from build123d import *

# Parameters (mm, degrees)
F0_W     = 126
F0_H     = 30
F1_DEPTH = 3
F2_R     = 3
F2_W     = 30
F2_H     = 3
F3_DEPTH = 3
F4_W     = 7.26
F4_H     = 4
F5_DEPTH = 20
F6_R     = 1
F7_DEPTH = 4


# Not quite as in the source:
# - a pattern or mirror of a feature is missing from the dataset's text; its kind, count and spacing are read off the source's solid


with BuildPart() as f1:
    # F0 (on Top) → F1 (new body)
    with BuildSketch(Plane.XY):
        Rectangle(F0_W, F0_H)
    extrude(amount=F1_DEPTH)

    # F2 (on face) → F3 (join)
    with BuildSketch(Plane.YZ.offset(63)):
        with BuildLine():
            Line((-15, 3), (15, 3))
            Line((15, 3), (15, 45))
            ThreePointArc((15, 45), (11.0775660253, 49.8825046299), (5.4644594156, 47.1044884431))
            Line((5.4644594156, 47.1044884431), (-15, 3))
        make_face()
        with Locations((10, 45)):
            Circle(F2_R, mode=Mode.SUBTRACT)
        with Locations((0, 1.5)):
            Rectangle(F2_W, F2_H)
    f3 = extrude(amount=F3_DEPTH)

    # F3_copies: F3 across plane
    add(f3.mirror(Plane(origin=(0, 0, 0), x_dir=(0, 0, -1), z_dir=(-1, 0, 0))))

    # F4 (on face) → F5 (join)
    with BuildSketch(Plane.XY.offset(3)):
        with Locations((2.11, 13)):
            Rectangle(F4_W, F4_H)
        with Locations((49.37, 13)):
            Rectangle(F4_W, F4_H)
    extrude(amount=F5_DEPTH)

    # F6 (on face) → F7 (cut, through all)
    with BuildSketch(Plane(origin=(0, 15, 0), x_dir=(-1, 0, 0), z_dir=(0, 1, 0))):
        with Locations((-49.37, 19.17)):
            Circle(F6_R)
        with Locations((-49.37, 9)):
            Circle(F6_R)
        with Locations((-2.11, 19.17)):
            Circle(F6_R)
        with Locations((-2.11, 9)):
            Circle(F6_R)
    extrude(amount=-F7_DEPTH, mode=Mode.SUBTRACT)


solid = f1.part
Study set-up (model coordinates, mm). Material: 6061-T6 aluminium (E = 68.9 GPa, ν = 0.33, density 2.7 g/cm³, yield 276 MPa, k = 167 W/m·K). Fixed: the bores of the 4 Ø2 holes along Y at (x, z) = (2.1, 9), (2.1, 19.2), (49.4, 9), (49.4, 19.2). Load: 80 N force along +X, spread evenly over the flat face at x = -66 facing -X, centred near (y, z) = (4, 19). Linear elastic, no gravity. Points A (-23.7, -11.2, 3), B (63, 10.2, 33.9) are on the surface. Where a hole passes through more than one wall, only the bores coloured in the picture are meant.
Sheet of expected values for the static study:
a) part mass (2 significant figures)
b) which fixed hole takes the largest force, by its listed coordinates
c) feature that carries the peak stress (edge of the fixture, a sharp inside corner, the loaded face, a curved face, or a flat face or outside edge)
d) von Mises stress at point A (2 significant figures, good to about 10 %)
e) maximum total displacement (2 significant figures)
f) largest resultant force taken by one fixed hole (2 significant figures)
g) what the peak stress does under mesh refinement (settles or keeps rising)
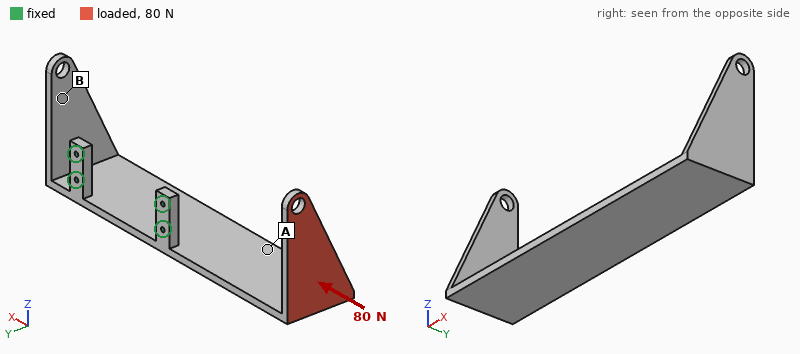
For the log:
49 g
(2.1, 9)
a sharp inside corner
31 MPa
1.4 mm
93 N
keeps rising
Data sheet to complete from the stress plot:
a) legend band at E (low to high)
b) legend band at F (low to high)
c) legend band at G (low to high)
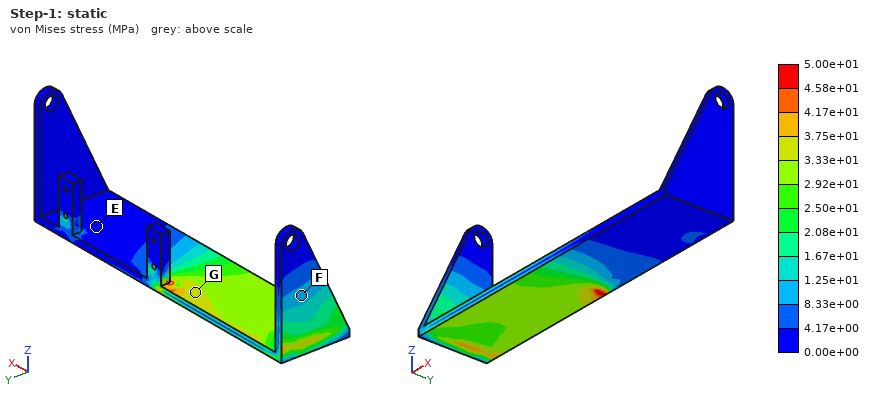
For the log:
0.00e+00 to 4.17e+00 MPa
8.33e+00 to 1.25e+01 MPa
3.33e+01 to 3.75e+01 MPa
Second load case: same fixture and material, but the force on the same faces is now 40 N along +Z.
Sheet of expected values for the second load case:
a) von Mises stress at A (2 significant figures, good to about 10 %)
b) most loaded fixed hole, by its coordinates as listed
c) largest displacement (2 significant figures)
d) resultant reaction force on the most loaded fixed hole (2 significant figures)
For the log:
36 MPa
(49.4, 9)
1.6 mm
130 N
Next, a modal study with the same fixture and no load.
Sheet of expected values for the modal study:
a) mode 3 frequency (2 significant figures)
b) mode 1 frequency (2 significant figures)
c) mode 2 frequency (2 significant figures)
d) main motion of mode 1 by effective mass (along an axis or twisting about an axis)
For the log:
950 Hz
270 Hz
650 Hz
along Z
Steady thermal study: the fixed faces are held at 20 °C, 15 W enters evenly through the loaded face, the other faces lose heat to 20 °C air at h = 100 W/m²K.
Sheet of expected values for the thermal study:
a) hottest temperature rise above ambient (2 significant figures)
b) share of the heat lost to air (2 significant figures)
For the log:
43 K
83 %
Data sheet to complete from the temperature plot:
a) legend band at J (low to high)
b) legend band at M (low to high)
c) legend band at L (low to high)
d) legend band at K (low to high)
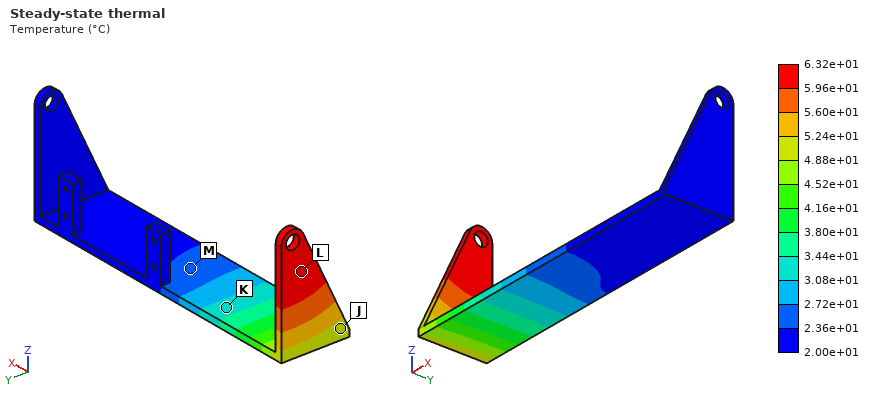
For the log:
4.88e+01 to 5.24e+01 °C
2.36e+01 to 2.72e+01 °C
5.96e+01 to 6.32e+01 °C
3.08e+01 to 3.44e+01 °C
